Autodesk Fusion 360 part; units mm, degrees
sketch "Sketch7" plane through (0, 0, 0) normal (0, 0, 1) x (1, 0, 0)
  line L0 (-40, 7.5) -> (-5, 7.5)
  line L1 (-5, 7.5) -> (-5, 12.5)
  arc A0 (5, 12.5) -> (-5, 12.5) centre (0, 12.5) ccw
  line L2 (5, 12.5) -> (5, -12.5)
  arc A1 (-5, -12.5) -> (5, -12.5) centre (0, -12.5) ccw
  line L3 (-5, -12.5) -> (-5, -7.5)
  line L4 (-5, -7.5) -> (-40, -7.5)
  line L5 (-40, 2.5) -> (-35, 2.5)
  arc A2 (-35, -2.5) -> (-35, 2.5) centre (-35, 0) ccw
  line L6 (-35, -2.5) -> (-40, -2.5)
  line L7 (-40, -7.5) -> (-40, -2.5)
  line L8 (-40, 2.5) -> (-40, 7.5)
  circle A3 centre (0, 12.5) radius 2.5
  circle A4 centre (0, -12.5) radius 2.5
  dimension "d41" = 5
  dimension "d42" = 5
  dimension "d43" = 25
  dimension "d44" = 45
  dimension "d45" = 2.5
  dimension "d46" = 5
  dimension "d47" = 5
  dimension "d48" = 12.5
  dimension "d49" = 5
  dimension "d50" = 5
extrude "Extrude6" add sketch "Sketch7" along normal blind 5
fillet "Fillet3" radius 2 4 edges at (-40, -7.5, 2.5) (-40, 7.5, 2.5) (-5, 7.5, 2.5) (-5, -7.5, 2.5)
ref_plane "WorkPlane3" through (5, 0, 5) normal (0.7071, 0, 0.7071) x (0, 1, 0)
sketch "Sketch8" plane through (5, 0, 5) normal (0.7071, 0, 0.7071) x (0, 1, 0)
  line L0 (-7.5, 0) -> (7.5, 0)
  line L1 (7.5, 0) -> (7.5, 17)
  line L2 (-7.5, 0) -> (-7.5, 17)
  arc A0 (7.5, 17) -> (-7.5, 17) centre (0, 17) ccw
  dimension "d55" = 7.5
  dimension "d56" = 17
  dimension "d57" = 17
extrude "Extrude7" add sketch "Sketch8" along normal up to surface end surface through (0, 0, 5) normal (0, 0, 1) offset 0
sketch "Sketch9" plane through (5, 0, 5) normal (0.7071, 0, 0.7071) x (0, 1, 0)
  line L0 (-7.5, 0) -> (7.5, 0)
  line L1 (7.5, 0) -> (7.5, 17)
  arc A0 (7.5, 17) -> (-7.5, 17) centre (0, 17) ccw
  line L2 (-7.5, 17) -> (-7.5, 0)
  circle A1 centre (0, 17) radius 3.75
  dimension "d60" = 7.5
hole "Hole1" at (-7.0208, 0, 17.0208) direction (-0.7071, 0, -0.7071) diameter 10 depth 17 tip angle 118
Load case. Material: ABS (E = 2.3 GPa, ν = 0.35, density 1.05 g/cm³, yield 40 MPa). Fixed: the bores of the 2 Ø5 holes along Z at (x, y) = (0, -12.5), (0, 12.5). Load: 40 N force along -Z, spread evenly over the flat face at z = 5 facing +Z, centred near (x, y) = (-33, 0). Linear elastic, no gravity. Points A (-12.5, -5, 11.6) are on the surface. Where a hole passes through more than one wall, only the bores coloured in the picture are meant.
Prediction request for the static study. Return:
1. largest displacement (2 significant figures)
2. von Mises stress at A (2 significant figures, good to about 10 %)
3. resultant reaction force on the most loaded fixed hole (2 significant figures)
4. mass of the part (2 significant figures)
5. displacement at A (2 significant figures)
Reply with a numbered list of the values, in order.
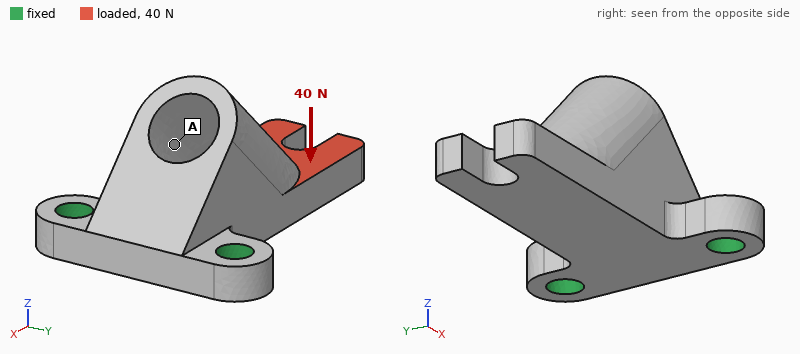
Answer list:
1. 0.61 mm
2. 2.5 MPa
3. 26 N
4. 6.8 g
5. 0.19 mm
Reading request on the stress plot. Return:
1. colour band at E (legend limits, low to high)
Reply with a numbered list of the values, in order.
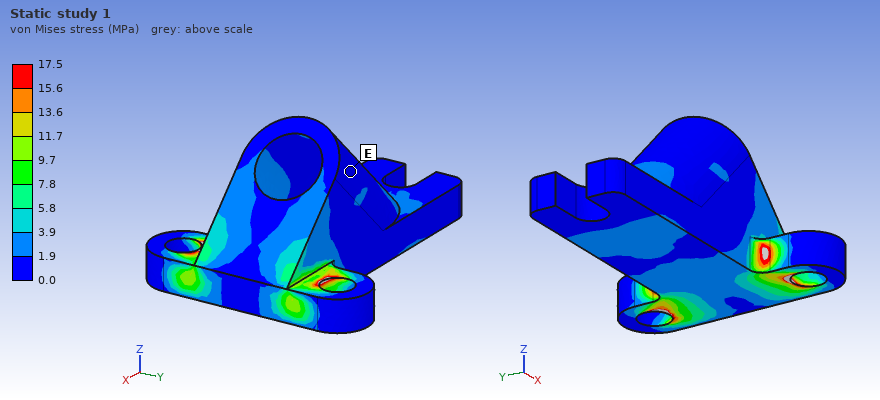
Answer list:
1. 0.0 to 1.9 MPa
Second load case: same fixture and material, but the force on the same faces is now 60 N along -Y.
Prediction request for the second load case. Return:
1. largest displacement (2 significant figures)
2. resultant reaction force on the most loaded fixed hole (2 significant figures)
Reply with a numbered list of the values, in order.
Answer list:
1. 0.22 mm
2. 94 N
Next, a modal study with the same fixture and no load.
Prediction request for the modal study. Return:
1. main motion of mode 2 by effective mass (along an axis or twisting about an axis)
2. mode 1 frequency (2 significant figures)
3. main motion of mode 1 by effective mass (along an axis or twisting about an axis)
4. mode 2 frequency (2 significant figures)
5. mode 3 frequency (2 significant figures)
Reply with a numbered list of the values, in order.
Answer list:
1. along Y
2. 1100 Hz
3. along Z
4. 2600 Hz
5. 4700 Hz
